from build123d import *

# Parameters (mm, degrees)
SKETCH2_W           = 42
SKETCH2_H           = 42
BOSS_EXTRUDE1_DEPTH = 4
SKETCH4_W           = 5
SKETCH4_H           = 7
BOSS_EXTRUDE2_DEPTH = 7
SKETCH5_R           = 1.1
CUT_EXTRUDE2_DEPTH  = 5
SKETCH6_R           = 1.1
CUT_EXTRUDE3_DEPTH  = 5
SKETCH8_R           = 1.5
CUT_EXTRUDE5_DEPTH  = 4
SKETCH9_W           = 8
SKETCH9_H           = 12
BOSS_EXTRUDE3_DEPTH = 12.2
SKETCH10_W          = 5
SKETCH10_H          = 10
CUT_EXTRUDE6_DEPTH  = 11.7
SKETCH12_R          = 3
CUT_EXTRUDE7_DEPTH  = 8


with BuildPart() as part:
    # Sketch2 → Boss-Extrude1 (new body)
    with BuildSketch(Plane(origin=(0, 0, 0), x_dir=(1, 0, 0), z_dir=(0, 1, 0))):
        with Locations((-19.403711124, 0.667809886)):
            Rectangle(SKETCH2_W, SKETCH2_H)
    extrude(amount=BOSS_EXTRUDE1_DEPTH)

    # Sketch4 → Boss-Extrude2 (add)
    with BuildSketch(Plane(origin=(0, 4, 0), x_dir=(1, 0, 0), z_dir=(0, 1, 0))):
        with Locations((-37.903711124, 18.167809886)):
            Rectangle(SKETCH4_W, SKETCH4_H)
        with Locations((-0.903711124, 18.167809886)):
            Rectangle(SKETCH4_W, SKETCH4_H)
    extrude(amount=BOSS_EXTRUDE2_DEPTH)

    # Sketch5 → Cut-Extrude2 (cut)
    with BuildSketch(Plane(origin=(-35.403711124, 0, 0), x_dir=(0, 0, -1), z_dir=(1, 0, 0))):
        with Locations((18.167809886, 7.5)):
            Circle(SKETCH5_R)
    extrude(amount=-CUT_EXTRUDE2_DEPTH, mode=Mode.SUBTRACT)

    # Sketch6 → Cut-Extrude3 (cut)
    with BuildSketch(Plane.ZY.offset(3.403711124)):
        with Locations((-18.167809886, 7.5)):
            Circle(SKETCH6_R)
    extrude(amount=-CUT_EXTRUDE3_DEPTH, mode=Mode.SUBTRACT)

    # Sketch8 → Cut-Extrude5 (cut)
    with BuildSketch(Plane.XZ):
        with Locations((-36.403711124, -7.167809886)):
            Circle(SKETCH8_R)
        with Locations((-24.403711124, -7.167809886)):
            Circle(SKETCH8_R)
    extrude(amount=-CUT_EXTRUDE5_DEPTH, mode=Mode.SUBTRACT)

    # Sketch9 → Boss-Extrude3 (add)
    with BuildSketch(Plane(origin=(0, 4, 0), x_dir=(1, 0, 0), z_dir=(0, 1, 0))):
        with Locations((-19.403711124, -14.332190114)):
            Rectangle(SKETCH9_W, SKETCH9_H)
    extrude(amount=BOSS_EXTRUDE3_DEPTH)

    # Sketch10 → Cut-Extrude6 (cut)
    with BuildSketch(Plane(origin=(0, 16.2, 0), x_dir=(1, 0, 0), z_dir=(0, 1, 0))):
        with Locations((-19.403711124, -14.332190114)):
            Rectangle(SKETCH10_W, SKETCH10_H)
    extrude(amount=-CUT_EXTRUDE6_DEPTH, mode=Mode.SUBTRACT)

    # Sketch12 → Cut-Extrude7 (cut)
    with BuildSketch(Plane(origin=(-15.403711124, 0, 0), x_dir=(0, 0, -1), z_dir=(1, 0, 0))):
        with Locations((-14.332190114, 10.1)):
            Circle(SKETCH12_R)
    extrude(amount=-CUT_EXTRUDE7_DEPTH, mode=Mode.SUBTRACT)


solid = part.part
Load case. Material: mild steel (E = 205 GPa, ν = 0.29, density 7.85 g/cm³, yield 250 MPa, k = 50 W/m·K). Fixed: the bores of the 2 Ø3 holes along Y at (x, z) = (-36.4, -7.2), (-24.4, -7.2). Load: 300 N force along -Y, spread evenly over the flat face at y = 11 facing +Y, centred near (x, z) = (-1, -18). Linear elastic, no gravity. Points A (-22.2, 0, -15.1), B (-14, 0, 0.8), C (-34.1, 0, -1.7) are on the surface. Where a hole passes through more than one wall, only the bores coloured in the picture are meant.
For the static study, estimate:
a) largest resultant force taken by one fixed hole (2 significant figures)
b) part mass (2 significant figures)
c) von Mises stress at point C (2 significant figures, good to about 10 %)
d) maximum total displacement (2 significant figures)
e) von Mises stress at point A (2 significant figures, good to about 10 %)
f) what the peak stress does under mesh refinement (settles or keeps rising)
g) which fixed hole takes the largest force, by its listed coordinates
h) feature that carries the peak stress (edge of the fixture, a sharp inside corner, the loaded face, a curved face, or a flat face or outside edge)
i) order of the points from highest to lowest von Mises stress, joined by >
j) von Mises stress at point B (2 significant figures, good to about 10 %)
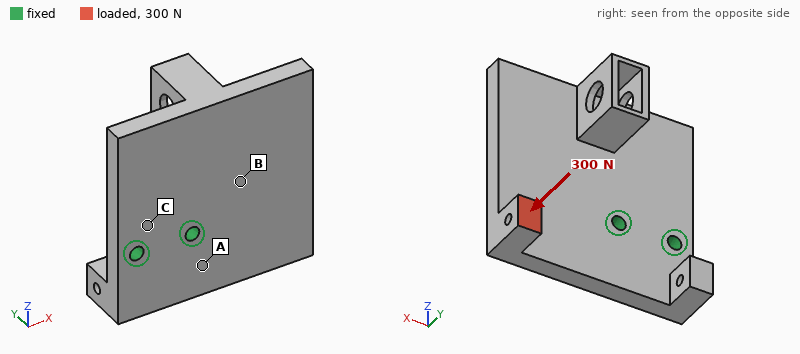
580 N
62 g
22 MPa
85 µm
71 MPa
keeps rising
(-24.4, -7.2)
edge of the fixture
A > B > C
44 MPa
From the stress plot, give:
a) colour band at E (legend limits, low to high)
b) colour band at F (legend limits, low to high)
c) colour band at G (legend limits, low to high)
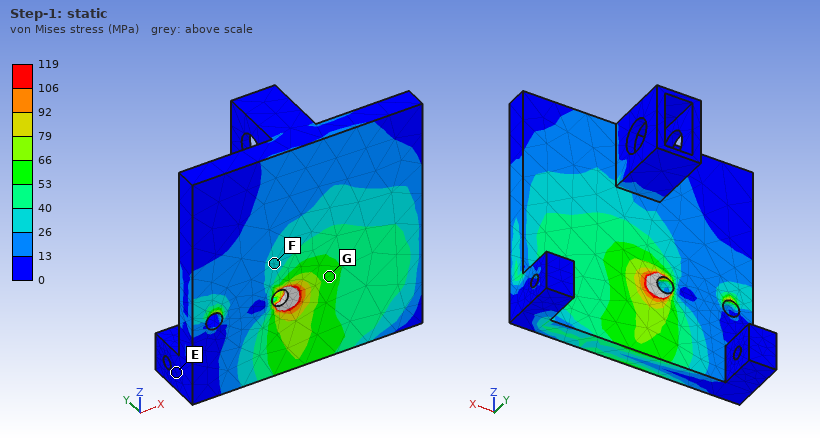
0 to 13 MPa
26 to 40 MPa
53 to 66 MPa
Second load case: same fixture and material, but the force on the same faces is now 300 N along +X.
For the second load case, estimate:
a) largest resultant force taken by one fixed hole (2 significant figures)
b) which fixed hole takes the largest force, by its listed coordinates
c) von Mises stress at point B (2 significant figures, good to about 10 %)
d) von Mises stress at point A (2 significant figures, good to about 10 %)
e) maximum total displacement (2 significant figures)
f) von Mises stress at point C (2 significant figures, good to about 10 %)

340 N
(-24.4, -7.2)
23 MPa
21 MPa
49 µm
9.3 MPa
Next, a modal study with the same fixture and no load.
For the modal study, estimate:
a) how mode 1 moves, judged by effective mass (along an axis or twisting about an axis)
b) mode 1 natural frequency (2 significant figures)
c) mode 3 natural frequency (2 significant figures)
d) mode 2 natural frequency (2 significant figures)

along Y
2800 Hz
6600 Hz
3900 Hz
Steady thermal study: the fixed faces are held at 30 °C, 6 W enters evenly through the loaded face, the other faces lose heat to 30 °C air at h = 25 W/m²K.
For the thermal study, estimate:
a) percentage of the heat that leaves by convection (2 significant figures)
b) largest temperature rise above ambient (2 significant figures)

21 %
66 K
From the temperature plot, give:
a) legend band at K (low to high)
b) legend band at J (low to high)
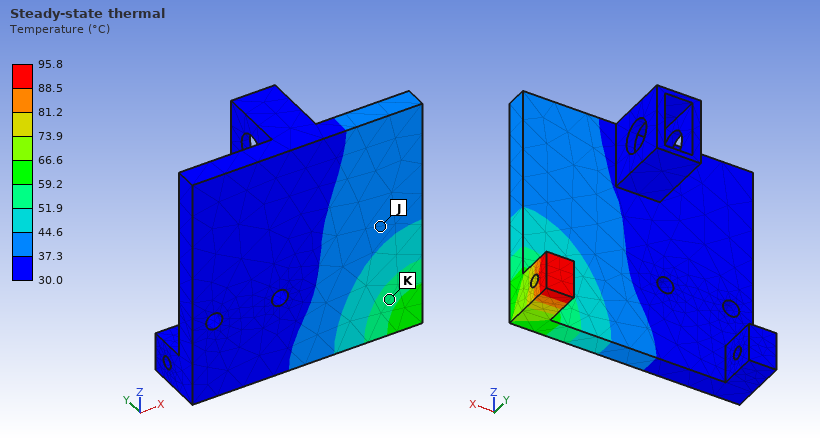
51.9 to 59.2 °C
37.3 to 44.6 °C
